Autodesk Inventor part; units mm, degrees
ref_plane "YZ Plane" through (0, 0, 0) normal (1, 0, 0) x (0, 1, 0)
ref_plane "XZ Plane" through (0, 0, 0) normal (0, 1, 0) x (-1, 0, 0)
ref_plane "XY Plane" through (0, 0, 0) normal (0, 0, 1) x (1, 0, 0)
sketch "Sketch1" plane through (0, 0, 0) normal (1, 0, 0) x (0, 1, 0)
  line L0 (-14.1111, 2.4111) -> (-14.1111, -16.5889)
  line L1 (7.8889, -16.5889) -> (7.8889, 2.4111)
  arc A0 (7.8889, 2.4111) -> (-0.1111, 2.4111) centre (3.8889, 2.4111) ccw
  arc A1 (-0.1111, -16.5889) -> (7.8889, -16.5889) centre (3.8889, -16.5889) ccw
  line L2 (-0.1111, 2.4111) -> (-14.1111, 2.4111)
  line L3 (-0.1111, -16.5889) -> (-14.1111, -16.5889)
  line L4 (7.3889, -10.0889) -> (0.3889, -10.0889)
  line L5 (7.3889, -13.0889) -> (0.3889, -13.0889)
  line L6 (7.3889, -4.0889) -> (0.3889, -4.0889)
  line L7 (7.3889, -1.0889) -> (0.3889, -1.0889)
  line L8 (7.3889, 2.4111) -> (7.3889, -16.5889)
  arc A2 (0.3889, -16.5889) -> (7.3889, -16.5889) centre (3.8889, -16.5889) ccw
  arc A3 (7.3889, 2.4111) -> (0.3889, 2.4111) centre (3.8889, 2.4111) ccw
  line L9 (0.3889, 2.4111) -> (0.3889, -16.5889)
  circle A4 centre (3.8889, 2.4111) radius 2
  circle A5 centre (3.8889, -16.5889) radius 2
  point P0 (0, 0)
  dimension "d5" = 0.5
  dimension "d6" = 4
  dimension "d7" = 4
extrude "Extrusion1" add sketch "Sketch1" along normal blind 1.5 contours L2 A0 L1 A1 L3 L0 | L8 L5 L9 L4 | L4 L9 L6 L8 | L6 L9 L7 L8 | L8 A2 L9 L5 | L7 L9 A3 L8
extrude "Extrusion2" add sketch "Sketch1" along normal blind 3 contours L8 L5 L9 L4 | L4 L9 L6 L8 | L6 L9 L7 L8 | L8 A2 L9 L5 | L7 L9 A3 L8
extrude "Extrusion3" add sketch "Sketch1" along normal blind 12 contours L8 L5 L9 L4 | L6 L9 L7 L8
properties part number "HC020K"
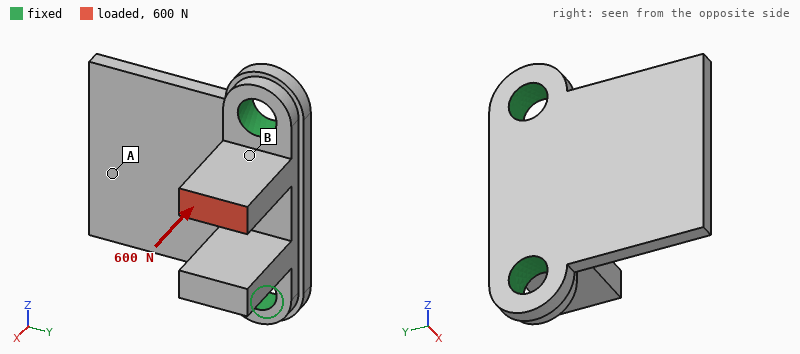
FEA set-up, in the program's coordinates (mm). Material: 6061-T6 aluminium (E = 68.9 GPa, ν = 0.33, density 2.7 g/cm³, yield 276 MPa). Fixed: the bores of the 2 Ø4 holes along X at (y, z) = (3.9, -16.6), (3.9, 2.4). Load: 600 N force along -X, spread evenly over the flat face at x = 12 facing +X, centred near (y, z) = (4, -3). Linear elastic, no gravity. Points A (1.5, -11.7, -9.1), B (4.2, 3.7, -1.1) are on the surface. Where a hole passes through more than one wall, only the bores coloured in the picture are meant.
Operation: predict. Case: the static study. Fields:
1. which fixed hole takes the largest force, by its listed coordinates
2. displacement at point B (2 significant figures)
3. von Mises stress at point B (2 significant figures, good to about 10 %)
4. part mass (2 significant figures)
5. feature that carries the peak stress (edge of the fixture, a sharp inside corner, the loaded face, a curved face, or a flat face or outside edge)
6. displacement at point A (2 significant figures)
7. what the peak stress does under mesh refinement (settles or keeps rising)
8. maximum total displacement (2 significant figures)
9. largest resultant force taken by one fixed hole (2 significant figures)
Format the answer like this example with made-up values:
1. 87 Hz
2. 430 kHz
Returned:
1. (3.9, 2.4)
2. 5.3 µm
3. 36 MPa
4. 3.4 g
5. edge of the fixture
6. 5.9 µm
7. keeps rising
8. 17 µm
9. 500 N
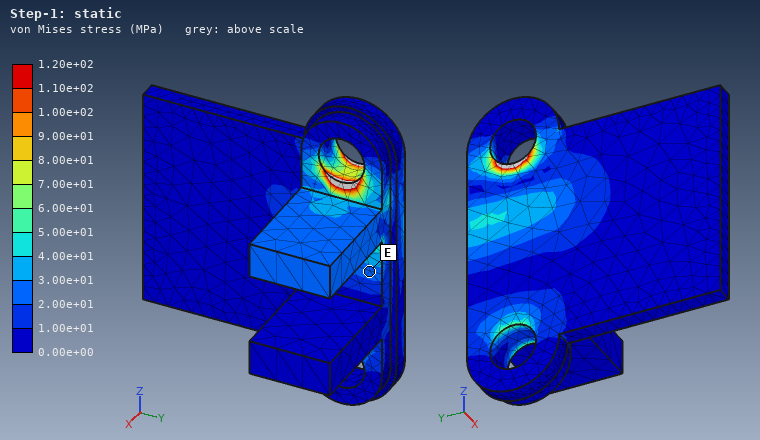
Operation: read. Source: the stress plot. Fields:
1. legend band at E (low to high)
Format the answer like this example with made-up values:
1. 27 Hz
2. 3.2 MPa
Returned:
1. 2.00e+01 to 3.00e+01 MPa
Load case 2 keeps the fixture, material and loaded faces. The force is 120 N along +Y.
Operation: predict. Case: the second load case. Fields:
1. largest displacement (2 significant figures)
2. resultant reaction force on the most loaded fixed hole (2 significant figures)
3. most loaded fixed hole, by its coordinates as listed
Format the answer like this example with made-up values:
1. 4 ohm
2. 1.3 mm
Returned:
1. 26 µm
2. 100 N
3. (3.9, 2.4)
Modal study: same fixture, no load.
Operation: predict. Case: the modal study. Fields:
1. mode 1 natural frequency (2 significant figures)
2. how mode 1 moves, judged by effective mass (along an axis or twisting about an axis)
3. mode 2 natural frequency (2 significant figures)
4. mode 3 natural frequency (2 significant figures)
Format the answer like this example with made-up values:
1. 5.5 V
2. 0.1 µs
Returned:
1. 5100 Hz
2. along X
3. 11 kHz
4. 18 kHz
